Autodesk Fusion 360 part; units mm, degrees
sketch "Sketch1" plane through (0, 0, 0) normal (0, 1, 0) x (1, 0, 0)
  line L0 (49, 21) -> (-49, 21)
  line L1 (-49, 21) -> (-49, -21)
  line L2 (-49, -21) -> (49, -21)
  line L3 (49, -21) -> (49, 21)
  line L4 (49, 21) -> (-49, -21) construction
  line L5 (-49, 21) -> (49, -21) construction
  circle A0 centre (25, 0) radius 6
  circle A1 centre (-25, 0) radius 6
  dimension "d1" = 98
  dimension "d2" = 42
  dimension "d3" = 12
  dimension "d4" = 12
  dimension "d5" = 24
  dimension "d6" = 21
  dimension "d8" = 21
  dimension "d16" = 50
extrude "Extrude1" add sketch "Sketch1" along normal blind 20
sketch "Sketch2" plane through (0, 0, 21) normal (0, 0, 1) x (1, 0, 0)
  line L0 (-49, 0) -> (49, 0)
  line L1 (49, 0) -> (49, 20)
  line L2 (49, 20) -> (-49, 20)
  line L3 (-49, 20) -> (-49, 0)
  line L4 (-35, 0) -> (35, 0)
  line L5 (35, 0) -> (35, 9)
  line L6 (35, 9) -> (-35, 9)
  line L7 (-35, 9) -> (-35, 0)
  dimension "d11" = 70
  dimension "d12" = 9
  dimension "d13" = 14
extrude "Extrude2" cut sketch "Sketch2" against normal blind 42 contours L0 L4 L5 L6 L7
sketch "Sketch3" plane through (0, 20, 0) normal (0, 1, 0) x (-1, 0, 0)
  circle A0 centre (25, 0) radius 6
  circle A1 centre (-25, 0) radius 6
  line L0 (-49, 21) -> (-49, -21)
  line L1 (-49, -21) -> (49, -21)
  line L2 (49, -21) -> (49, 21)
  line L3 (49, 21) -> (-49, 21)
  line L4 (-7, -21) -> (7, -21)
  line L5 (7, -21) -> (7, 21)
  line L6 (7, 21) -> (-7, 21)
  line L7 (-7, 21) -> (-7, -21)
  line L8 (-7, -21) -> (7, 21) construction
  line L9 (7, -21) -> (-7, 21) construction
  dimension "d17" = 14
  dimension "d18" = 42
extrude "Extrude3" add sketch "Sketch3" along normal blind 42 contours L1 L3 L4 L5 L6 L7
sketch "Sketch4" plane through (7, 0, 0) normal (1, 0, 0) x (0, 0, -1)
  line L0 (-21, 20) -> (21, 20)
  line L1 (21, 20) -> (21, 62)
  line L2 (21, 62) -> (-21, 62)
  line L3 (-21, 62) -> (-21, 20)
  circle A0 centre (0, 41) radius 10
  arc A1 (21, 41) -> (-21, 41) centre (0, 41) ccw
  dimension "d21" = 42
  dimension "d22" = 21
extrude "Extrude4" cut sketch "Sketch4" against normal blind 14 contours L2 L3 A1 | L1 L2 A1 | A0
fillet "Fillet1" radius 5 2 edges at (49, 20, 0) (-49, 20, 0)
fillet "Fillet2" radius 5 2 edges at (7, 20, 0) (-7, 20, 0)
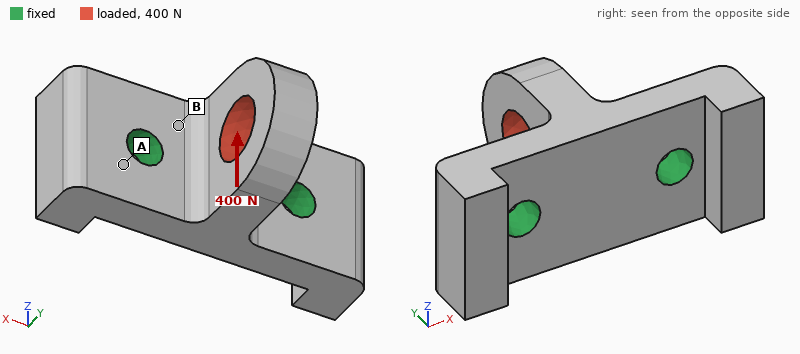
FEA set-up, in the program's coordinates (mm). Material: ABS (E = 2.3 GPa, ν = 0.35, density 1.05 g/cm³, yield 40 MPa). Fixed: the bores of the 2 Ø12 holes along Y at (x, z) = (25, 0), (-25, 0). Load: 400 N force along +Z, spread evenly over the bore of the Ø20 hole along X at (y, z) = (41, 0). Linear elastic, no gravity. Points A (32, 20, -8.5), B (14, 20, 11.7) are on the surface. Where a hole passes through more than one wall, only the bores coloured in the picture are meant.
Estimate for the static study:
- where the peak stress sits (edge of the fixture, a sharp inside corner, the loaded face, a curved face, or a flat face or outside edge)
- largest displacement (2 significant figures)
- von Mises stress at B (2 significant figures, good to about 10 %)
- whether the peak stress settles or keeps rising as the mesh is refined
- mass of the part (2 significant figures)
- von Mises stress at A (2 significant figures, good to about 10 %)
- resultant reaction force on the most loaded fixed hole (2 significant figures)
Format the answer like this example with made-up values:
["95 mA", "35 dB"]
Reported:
["edge of the fixture", "0.29 mm", "3.5 MPa", "keeps rising", "75 g", "1.2 MPa", "200 N"]
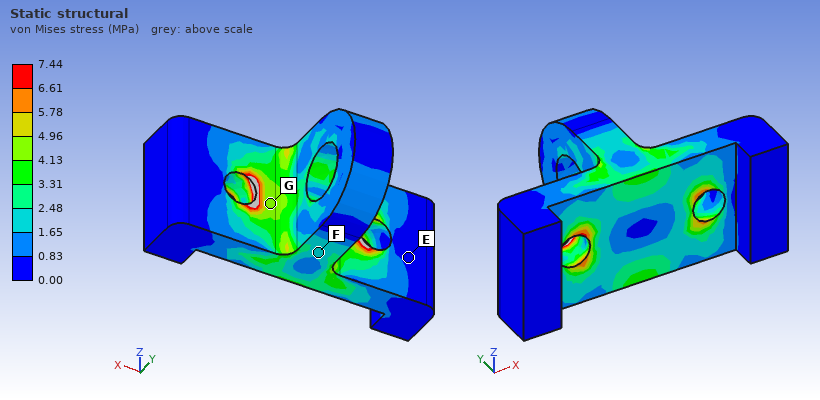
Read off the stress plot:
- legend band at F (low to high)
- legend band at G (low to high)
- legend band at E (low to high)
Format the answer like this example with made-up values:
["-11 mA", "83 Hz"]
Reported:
["1.65 to 2.48 MPa", "4.13 to 4.96 MPa", "0.00 to 0.83 MPa"]
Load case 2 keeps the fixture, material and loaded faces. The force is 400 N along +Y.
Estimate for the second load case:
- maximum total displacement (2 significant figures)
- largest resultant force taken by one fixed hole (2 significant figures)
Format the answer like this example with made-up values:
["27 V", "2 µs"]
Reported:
["42 µm", "210 N"]
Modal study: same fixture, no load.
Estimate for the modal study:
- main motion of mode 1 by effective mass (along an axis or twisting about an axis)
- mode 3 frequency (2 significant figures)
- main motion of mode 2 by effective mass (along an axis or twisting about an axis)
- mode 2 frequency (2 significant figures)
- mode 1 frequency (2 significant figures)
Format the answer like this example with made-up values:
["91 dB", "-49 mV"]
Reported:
["along Z", "3100 Hz", "along X", "1700 Hz", "1600 Hz"]
